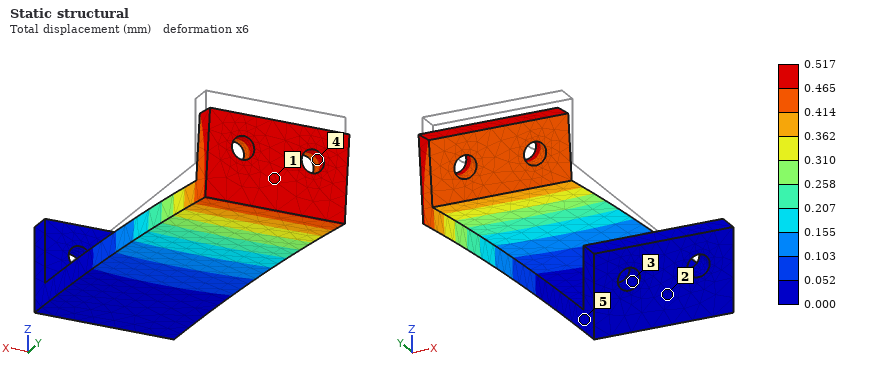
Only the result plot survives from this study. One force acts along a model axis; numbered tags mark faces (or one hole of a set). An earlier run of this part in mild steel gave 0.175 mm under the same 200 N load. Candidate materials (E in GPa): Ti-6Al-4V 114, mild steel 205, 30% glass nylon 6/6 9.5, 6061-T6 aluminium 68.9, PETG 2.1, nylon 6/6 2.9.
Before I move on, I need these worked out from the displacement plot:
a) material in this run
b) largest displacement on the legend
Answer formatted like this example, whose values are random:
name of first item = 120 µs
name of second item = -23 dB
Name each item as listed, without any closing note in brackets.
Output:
material in this run = 6061-T6 aluminium
largest displacement on the legend = 0.517 mm
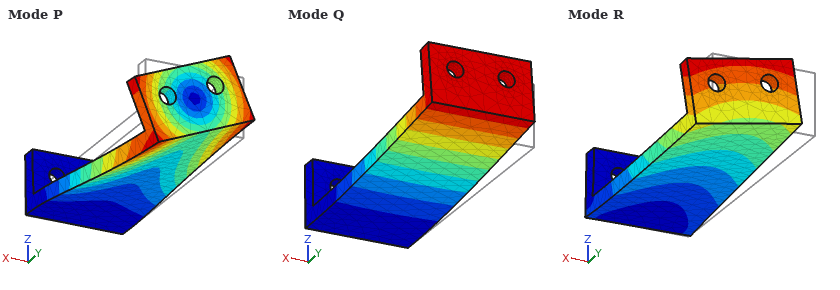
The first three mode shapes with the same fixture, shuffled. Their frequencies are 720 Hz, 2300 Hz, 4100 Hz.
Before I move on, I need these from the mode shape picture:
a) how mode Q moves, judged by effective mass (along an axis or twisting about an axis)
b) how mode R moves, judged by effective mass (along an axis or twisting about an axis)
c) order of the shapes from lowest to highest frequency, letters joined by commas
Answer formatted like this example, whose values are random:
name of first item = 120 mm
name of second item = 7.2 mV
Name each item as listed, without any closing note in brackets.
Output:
how mode Q moves, judged by effective mass = along Z
how mode R moves, judged by effective mass = along X
order of the shapes from lowest to highest frequency, letters joined by commas = Q, R, P
